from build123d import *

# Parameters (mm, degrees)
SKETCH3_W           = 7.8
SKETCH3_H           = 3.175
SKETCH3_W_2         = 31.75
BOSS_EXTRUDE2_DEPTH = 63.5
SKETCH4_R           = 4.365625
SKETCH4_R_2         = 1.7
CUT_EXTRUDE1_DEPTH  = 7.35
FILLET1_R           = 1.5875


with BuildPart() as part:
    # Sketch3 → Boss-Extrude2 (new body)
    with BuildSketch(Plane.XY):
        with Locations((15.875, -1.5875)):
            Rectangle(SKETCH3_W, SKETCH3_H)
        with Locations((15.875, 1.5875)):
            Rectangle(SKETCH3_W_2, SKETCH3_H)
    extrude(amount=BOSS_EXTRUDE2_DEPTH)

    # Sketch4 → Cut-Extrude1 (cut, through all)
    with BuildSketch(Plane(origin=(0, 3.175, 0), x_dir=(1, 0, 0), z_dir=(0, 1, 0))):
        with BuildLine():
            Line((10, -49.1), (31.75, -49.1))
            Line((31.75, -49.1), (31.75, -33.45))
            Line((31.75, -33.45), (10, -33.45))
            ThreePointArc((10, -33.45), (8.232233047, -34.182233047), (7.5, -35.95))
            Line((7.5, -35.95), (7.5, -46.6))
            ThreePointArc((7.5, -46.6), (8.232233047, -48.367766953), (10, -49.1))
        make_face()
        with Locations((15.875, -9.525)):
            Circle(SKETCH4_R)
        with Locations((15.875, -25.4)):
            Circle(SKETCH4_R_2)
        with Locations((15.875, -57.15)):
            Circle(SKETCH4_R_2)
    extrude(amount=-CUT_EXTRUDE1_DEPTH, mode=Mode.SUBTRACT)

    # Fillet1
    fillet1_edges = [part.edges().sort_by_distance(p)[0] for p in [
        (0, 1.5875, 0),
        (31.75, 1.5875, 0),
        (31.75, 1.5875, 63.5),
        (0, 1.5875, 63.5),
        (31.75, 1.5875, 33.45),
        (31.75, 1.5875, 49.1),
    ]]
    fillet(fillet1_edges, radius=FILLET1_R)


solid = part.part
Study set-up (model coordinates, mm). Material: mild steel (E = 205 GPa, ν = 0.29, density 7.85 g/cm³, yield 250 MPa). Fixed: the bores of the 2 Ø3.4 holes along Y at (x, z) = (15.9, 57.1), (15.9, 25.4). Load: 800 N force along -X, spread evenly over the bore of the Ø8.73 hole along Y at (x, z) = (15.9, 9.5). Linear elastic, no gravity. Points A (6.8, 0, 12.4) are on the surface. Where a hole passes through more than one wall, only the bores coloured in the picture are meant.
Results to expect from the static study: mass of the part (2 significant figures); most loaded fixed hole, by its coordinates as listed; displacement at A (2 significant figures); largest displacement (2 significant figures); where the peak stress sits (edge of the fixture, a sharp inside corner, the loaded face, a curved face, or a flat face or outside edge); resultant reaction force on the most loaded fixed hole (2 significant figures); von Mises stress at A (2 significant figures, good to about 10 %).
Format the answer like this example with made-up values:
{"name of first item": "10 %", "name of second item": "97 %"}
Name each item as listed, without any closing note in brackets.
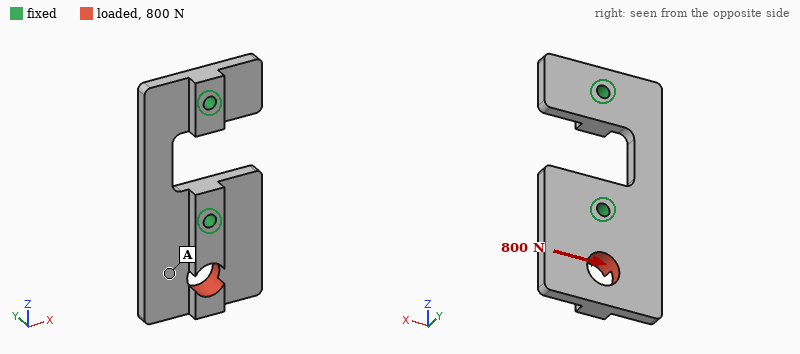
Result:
{"mass of the part": "46 g", "most loaded fixed hole, by its coordinates as listed": "(15.9, 25.4)", "displacement at A": "7.2 µm", "largest displacement": "15 µm", "where the peak stress sits": "edge of the fixture", "resultant reaction force on the most loaded fixed hole": "990 N", "von Mises stress at A": "18 MPa"}
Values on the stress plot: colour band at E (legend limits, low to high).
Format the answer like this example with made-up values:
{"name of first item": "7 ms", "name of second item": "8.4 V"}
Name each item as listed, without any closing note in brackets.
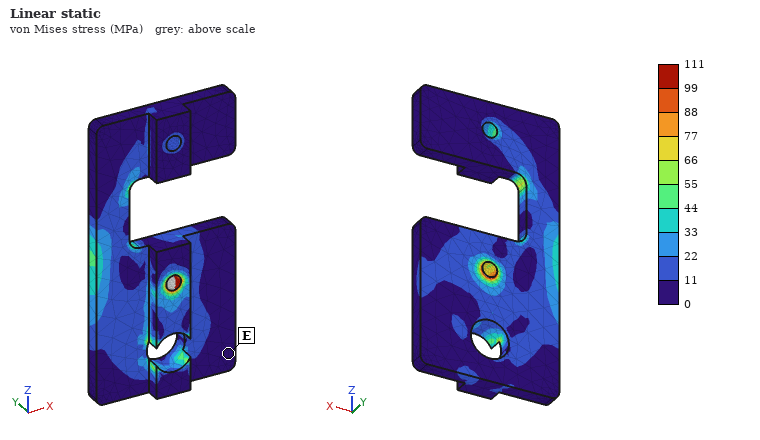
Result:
{"colour band at E": "0 to 11 MPa"}
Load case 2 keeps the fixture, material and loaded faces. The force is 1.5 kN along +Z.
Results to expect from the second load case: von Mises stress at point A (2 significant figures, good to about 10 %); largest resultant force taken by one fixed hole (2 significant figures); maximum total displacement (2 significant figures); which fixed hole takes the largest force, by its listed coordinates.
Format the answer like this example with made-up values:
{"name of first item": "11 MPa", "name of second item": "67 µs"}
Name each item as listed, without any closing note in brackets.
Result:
{"von Mises stress at point A": "32 MPa", "largest resultant force taken by one fixed hole": "1.5 kN", "maximum total displacement": "16 µm", "which fixed hole takes the largest force, by its listed coordinates": "(15.9, 25.4)"}
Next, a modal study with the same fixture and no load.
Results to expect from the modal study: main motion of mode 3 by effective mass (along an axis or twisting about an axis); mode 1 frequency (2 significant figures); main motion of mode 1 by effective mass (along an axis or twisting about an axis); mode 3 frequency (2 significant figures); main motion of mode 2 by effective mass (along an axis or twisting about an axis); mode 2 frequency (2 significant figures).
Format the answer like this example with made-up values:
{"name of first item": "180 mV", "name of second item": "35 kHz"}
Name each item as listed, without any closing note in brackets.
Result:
{"main motion of mode 3 by effective mass": "along X", "mode 1 frequency": "5200 Hz", "main motion of mode 1 by effective mass": "along Y", "mode 3 frequency": "9900 Hz", "main motion of mode 2 by effective mass": "twisting about Z", "mode 2 frequency": "7000 Hz"}
